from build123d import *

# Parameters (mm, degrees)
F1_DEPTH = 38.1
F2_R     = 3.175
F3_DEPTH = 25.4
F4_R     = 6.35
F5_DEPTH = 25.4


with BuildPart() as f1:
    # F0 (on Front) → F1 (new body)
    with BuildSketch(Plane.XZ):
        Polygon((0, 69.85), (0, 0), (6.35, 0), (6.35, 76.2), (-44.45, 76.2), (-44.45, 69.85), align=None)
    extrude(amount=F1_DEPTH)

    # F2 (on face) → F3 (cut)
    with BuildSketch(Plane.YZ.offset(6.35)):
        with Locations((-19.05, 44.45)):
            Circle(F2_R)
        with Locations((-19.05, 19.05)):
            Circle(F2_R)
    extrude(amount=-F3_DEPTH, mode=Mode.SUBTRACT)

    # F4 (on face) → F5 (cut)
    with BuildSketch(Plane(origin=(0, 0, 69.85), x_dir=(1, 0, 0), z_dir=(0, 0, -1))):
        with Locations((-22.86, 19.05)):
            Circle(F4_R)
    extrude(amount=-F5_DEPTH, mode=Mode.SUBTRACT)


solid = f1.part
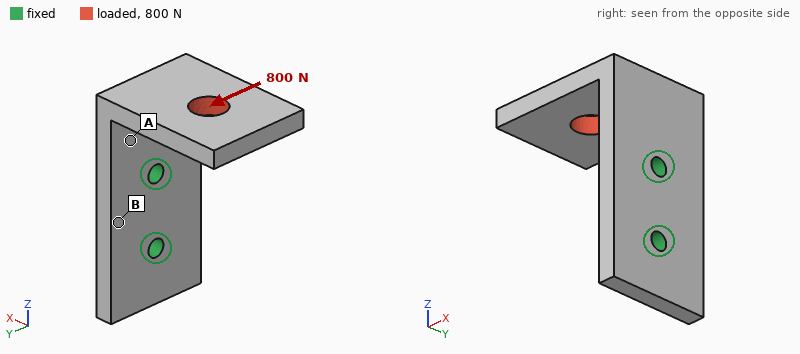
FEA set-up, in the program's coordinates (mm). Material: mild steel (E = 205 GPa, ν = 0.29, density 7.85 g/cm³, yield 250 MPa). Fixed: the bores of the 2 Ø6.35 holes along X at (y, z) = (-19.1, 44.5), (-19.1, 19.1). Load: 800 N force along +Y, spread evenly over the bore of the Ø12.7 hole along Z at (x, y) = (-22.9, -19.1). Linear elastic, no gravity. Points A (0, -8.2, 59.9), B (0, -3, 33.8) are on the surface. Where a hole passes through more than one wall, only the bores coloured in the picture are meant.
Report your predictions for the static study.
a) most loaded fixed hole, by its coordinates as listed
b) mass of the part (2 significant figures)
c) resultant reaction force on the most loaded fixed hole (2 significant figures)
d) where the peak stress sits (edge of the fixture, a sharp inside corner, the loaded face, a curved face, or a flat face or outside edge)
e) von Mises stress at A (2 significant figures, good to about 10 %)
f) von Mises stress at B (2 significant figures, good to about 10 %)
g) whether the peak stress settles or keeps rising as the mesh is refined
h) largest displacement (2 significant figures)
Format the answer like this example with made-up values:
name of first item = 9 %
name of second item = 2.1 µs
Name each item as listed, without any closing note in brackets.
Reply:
most loaded fixed hole, by its coordinates as listed = (-19.1, 44.5)
mass of the part = 220 g
resultant reaction force on the most loaded fixed hole = 1.4 kN
where the peak stress sits = edge of the fixture
von Mises stress at A = 60 MPa
von Mises stress at B = 16 MPa
whether the peak stress settles or keeps rising as the mesh is refined = keeps rising
largest displacement = 0.12 mm
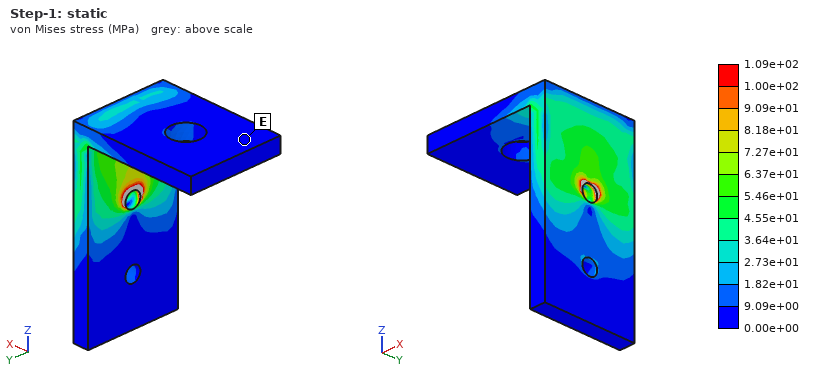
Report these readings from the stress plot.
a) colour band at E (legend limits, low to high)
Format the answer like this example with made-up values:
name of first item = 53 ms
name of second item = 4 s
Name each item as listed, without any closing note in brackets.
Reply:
colour band at E = 0.00e+00 to 9.09e+00 MPa
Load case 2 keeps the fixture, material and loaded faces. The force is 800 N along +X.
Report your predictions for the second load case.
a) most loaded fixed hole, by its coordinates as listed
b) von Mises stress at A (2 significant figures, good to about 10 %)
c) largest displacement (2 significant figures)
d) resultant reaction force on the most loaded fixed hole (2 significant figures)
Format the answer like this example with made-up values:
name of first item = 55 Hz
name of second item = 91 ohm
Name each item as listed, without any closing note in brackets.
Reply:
most loaded fixed hole, by its coordinates as listed = (-19.1, 44.5)
von Mises stress at A = 38 MPa
largest displacement = 0.11 mm
resultant reaction force on the most loaded fixed hole = 1.1 kN
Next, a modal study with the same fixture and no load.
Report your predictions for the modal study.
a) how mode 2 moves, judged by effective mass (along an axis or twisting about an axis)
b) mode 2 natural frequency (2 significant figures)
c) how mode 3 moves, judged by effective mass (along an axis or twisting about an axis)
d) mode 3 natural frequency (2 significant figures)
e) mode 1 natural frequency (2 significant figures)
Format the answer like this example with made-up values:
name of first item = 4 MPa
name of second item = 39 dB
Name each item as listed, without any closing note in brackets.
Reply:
how mode 2 moves, judged by effective mass = along Y
mode 2 natural frequency = 1700 Hz
how mode 3 moves, judged by effective mass = along X
mode 3 natural frequency = 3500 Hz
mode 1 natural frequency = 1200 Hz
